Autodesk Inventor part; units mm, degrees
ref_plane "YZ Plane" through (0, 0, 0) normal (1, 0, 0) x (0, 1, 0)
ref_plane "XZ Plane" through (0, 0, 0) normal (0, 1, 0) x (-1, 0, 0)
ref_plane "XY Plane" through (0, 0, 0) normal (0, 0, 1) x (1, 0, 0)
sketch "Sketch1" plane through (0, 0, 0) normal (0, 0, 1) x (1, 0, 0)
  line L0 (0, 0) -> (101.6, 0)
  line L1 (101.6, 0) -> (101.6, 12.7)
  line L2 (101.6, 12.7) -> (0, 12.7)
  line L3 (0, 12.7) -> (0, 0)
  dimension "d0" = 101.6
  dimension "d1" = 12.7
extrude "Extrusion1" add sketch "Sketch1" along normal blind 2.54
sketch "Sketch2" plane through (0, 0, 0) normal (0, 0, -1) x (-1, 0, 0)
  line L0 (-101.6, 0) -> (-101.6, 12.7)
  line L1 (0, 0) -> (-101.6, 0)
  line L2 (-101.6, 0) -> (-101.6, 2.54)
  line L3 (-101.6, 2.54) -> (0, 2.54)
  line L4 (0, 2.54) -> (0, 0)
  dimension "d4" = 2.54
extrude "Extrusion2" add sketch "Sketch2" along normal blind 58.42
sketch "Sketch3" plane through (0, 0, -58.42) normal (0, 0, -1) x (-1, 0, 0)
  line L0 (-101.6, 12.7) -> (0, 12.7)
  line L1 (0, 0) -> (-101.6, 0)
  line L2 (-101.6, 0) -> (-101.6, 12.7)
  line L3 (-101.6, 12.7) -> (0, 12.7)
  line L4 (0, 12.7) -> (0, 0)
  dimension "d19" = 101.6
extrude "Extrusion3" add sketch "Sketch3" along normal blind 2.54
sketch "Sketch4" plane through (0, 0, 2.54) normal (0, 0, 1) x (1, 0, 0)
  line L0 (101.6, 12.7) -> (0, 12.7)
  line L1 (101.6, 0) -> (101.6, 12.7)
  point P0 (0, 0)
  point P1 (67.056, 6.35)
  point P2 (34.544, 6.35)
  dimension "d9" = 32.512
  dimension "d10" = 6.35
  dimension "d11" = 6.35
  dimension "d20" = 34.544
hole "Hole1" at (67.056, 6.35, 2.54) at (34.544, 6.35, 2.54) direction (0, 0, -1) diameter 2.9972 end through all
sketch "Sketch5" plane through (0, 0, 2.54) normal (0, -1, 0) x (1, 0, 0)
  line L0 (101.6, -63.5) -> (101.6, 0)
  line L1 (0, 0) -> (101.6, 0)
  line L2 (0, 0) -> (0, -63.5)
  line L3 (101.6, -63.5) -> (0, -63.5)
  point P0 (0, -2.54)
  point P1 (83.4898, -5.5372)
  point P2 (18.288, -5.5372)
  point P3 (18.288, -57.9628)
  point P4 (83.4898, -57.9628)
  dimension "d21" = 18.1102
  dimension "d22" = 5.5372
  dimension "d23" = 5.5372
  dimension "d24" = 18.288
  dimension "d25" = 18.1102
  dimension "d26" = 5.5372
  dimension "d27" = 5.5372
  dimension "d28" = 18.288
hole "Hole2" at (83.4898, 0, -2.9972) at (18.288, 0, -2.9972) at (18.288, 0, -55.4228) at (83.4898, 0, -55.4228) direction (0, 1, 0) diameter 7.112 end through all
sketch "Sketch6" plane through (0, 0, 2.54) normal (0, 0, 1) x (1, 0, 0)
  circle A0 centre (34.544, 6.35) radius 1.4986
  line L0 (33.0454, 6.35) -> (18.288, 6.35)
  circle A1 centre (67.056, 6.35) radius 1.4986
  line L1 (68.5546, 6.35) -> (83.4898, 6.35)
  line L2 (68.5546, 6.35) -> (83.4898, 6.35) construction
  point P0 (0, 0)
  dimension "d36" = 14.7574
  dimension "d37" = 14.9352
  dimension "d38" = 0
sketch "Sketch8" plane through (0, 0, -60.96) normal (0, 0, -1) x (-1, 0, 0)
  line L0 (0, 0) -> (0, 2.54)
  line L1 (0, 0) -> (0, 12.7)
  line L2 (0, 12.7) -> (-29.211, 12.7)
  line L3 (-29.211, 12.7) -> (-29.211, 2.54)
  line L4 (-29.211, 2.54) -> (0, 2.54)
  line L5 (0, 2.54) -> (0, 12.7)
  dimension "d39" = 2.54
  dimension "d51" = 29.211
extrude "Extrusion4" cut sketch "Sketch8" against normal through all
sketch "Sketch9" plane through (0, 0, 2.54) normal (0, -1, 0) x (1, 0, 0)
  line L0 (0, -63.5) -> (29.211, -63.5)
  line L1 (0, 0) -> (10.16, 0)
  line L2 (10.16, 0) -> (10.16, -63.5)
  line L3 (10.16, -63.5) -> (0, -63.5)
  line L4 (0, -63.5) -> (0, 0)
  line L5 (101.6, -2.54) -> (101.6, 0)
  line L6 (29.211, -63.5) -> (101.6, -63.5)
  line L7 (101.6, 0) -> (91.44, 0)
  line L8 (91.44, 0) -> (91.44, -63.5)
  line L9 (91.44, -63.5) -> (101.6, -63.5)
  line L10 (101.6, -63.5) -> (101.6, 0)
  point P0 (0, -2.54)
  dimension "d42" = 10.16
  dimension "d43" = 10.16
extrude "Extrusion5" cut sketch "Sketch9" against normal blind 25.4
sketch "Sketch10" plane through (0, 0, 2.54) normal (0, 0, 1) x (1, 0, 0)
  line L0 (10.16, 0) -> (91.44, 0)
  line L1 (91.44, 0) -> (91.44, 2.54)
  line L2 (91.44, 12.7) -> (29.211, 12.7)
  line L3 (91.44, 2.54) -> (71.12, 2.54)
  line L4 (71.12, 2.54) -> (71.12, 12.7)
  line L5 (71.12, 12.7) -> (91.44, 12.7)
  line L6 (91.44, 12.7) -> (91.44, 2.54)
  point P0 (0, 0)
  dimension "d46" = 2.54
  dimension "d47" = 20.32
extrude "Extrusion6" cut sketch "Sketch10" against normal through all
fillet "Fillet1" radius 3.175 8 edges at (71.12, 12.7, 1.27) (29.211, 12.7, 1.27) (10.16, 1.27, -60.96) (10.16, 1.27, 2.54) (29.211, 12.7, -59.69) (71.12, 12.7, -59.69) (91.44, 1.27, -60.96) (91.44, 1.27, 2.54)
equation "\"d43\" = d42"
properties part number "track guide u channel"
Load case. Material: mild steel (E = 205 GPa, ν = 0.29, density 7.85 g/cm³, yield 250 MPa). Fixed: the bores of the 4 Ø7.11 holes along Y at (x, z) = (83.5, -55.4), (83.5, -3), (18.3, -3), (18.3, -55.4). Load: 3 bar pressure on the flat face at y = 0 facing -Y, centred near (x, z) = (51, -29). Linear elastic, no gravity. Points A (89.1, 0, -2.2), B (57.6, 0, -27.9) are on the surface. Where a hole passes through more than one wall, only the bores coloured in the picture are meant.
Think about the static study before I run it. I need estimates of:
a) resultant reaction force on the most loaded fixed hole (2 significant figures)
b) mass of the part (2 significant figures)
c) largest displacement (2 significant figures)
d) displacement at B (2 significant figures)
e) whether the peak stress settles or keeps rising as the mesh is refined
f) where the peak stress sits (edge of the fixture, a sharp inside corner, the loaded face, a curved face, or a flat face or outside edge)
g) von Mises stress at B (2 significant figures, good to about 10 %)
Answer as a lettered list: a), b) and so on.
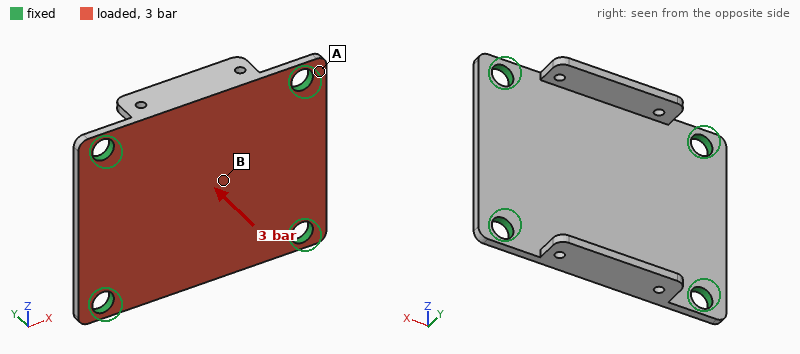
a) 390 N
b) 120 g
c) 53 µm
d) 51 µm
e) keeps rising
f) edge of the fixture
g) 41 MPa
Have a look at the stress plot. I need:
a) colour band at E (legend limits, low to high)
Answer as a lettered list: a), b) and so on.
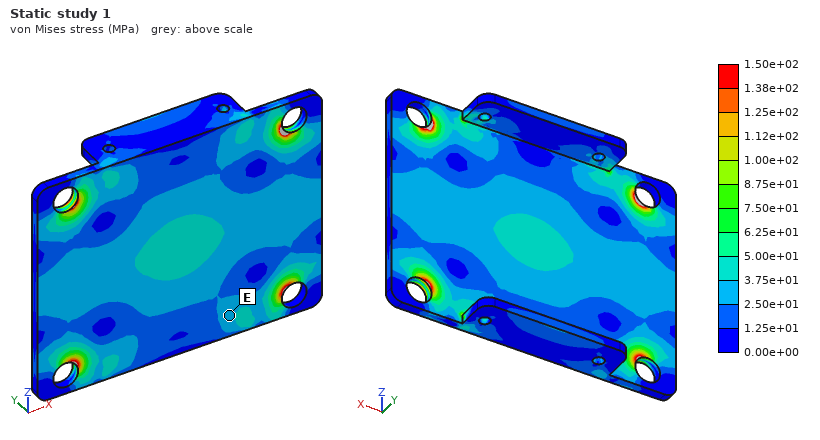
a) 2.50e+01 to 3.75e+01 MPa
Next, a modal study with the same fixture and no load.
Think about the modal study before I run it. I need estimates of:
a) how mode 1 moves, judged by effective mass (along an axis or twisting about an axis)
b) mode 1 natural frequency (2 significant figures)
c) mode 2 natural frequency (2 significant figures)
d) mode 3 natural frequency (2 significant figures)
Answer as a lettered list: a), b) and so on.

a) along Y
b) 3300 Hz
c) 5800 Hz
d) 5900 Hz
